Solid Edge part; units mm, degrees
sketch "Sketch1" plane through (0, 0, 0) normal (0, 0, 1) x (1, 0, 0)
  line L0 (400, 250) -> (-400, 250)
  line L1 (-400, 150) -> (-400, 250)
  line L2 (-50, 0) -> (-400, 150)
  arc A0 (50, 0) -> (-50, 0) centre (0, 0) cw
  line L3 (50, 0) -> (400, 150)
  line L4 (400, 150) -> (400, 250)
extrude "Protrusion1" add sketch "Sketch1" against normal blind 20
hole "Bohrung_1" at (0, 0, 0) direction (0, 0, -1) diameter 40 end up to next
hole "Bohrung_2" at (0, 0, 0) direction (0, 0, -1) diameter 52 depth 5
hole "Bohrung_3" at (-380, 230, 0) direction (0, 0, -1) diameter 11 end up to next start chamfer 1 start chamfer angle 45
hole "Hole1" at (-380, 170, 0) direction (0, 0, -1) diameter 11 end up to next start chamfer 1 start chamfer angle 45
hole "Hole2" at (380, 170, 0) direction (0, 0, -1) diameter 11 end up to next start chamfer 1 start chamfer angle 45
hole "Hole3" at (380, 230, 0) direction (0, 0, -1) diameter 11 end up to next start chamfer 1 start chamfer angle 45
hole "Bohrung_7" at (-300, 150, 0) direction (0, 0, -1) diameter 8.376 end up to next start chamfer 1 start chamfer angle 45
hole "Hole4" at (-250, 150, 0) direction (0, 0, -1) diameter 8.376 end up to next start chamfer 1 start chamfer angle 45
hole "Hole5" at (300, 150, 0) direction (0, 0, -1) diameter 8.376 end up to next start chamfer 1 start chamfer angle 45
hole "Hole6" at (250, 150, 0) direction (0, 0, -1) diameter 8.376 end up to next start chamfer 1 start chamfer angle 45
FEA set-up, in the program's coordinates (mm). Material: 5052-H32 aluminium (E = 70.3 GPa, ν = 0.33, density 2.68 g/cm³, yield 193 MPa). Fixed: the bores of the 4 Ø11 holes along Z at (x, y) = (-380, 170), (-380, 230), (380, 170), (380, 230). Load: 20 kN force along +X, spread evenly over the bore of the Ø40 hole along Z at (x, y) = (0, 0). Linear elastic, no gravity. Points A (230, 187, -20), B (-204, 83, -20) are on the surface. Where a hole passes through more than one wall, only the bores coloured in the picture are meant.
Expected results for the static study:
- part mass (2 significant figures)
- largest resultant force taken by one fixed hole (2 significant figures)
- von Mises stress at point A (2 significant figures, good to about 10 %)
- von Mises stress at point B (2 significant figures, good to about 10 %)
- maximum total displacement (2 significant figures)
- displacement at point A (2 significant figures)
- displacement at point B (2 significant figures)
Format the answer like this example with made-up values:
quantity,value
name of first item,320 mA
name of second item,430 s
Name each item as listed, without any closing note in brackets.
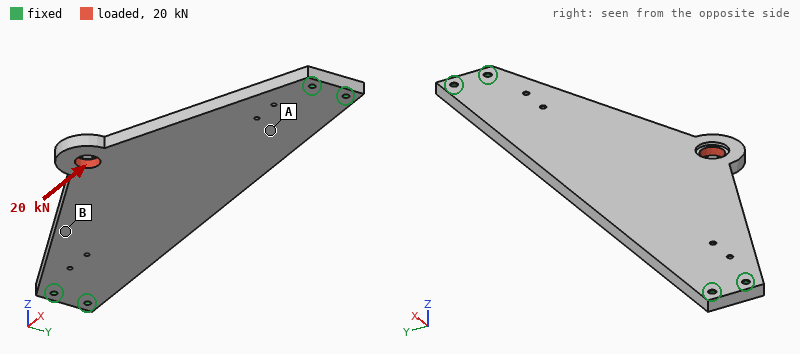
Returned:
quantity,value
part mass,8.0 kg
largest resultant force taken by one fixed hole,6.9 kN
von Mises stress at point A,3.1 MPa
von Mises stress at point B,7.7 MPa
maximum total displacement,73 µm
displacement at point A,17 µm
displacement at point B,29 µm
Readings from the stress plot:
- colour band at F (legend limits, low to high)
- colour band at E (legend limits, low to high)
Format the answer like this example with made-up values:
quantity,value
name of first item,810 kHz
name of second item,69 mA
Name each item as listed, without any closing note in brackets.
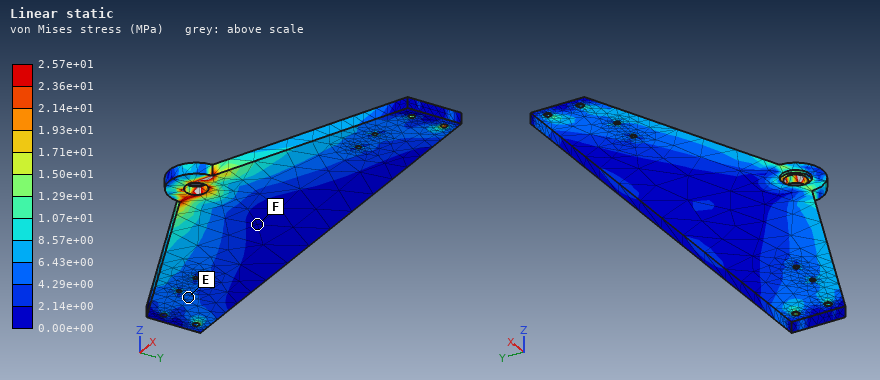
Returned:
quantity,value
colour band at F,0.00e+00 to 2.14e+00 MPa
colour band at E,4.29e+00 to 6.43e+00 MPa
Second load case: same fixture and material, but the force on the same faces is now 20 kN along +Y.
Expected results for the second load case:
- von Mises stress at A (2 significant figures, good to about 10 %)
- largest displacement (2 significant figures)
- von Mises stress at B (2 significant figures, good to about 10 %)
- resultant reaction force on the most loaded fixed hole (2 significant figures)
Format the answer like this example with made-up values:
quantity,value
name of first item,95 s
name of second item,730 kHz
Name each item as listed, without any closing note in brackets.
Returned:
quantity,value
von Mises stress at A,7.5 MPa
largest displacement,0.26 mm
von Mises stress at B,11 MPa
resultant reaction force on the most loaded fixed hole,16 kN
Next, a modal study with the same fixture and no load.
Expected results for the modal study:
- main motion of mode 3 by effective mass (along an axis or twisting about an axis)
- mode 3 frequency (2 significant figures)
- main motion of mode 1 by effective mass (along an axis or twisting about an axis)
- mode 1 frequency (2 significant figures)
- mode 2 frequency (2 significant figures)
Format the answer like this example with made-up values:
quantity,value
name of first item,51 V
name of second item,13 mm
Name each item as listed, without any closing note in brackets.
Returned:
quantity,value
main motion of mode 3 by effective mass,twisting about Y
mode 3 frequency,440 Hz
main motion of mode 1 by effective mass,along Z
mode 1 frequency,140 Hz
mode 2 frequency,300 Hz
